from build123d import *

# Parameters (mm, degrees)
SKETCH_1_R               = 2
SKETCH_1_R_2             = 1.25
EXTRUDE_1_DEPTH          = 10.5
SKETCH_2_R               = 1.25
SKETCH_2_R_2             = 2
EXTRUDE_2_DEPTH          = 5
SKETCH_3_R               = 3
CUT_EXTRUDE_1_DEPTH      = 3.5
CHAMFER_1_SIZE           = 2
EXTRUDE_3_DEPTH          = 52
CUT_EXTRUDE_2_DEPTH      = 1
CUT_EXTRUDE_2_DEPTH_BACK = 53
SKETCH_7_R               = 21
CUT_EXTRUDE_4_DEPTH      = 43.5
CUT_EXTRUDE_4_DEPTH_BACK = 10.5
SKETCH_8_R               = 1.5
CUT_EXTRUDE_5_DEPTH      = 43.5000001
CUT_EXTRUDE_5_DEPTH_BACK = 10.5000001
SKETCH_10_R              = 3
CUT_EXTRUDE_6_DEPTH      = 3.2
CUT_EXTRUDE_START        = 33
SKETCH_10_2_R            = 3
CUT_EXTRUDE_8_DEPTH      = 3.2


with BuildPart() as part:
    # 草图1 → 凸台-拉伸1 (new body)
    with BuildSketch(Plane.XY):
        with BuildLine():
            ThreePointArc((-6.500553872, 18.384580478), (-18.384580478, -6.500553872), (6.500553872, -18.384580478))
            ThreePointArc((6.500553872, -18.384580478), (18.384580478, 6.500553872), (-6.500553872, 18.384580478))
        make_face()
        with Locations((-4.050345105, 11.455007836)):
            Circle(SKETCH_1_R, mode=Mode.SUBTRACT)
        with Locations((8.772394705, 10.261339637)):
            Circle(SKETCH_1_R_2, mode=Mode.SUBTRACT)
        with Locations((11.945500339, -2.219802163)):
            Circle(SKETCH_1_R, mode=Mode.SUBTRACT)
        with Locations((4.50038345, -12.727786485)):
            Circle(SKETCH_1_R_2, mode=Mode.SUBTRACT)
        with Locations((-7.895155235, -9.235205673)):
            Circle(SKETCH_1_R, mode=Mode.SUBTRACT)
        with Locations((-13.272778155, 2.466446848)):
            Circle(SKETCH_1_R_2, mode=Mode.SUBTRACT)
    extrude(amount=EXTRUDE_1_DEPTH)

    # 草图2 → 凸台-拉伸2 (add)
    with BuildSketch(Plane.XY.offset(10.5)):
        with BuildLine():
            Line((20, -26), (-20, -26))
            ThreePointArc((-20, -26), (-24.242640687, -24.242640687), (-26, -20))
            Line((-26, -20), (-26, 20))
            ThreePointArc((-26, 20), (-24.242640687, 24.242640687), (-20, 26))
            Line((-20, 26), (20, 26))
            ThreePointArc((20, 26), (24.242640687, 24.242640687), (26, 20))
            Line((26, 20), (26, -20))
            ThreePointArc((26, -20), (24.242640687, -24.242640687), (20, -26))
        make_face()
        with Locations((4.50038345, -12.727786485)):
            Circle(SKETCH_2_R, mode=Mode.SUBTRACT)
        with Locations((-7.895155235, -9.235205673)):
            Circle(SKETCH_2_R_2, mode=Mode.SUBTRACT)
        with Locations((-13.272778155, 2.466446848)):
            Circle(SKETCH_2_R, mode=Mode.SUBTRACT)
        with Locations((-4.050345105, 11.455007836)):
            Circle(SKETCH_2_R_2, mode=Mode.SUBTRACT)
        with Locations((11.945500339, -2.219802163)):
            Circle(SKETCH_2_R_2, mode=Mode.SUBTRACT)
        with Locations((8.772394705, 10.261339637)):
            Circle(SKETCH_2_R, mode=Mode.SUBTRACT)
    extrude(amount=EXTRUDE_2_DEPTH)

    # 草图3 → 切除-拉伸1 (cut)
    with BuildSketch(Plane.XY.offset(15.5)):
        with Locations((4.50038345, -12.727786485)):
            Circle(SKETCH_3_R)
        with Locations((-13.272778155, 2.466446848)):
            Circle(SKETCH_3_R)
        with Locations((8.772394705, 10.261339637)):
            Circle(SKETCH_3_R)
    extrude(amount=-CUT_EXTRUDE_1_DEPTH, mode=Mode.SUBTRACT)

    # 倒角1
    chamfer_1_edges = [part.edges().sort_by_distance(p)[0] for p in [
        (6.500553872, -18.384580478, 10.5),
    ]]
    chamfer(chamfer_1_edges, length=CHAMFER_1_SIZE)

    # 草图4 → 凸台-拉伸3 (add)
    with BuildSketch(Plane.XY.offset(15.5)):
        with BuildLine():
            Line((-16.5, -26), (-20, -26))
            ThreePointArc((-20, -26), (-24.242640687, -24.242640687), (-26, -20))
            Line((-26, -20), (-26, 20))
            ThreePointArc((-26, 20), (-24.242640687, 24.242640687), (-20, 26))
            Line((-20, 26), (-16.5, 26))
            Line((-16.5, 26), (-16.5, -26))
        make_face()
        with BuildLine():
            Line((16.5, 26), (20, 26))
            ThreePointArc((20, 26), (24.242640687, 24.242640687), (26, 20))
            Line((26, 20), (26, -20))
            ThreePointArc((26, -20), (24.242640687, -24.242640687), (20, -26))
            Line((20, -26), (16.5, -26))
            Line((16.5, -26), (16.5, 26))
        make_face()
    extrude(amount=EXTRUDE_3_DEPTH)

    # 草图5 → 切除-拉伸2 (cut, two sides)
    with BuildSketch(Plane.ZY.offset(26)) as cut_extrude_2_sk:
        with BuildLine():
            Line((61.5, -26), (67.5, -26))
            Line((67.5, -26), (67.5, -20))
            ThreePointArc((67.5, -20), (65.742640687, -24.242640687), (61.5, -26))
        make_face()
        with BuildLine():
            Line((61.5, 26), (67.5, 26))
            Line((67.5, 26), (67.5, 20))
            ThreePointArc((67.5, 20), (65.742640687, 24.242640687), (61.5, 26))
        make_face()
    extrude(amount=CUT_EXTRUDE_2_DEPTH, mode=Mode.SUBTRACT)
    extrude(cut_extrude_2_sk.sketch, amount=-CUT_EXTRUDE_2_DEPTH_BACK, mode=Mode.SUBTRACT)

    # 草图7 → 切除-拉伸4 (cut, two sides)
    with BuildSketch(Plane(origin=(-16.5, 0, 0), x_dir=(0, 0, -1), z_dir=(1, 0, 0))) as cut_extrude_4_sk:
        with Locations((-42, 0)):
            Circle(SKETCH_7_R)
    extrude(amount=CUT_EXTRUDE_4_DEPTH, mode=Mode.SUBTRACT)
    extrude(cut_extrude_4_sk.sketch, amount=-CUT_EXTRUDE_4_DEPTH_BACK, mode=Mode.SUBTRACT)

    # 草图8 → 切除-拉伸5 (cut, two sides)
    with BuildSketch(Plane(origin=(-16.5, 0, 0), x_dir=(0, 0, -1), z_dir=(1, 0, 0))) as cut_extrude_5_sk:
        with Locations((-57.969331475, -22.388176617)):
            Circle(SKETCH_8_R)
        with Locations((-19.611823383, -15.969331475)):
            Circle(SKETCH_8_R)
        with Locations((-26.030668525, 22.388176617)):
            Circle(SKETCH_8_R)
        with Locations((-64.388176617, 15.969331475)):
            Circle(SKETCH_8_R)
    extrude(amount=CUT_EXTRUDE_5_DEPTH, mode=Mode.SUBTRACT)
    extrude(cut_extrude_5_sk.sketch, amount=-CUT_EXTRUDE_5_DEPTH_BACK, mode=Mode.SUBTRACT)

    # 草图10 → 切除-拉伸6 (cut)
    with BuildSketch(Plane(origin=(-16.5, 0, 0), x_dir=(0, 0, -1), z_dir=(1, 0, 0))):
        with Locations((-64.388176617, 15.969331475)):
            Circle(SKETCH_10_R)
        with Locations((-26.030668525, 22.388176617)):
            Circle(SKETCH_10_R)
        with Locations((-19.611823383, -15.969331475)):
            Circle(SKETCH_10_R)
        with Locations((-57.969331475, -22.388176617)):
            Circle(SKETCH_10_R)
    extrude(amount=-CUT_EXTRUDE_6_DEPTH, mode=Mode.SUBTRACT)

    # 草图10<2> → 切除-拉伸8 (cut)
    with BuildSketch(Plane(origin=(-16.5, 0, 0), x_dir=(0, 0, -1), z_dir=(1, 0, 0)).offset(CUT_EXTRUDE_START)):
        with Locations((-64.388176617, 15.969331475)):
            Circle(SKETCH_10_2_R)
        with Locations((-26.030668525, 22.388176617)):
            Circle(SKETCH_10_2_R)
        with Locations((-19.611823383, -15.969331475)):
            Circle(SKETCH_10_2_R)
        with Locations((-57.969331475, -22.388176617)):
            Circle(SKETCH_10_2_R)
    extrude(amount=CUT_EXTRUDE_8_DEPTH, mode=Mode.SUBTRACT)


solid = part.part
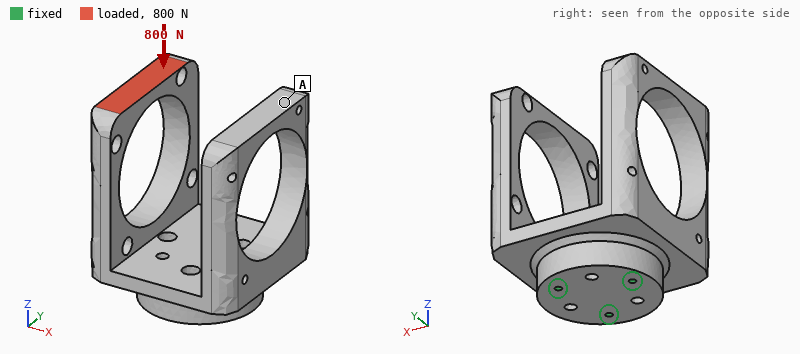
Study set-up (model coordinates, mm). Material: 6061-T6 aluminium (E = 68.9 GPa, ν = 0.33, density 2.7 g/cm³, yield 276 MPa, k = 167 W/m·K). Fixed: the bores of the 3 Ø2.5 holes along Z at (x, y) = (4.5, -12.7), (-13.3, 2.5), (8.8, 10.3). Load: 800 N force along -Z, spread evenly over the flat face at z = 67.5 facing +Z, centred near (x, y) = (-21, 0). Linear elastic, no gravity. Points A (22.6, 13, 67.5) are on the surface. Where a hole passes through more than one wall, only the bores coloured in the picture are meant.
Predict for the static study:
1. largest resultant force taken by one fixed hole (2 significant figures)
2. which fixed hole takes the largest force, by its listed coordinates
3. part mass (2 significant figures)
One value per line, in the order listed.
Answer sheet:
870 N
(-13.3, 2.5)
130 g
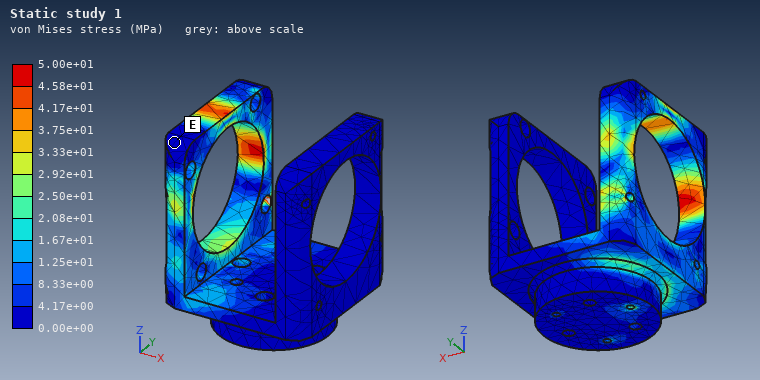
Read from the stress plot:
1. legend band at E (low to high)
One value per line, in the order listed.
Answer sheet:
0.00e+00 to 4.17e+00 MPa
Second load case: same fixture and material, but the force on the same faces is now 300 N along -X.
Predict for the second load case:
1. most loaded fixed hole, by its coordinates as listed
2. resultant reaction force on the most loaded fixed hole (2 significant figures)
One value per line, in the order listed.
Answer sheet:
(-13.3, 2.5)
760 N
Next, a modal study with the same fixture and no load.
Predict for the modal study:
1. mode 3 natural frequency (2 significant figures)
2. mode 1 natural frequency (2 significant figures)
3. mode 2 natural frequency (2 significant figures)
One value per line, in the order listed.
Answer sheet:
2500 Hz
1500 Hz
1500 Hz
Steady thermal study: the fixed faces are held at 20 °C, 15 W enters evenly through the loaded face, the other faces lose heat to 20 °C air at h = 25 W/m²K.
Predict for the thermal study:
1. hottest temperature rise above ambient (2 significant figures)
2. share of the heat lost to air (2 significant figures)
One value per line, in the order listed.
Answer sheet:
40 K
18 %
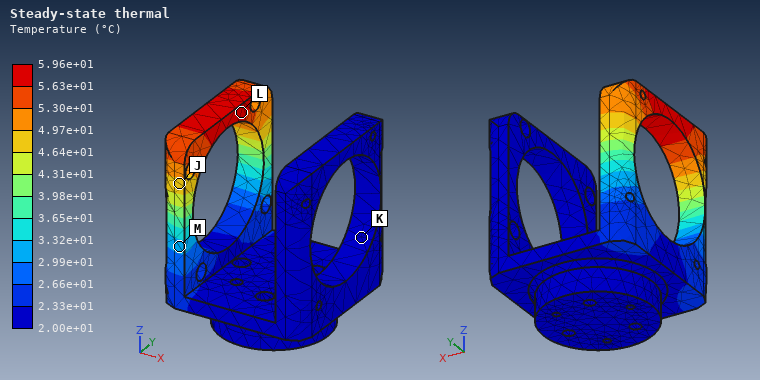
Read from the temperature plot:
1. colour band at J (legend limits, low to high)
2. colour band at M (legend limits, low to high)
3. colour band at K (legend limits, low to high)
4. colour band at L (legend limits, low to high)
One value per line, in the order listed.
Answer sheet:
4.64e+01 to 4.97e+01 °C
2.99e+01 to 3.32e+01 °C
2.00e+01 to 2.33e+01 °C
5.63e+01 to 5.96e+01 °C
